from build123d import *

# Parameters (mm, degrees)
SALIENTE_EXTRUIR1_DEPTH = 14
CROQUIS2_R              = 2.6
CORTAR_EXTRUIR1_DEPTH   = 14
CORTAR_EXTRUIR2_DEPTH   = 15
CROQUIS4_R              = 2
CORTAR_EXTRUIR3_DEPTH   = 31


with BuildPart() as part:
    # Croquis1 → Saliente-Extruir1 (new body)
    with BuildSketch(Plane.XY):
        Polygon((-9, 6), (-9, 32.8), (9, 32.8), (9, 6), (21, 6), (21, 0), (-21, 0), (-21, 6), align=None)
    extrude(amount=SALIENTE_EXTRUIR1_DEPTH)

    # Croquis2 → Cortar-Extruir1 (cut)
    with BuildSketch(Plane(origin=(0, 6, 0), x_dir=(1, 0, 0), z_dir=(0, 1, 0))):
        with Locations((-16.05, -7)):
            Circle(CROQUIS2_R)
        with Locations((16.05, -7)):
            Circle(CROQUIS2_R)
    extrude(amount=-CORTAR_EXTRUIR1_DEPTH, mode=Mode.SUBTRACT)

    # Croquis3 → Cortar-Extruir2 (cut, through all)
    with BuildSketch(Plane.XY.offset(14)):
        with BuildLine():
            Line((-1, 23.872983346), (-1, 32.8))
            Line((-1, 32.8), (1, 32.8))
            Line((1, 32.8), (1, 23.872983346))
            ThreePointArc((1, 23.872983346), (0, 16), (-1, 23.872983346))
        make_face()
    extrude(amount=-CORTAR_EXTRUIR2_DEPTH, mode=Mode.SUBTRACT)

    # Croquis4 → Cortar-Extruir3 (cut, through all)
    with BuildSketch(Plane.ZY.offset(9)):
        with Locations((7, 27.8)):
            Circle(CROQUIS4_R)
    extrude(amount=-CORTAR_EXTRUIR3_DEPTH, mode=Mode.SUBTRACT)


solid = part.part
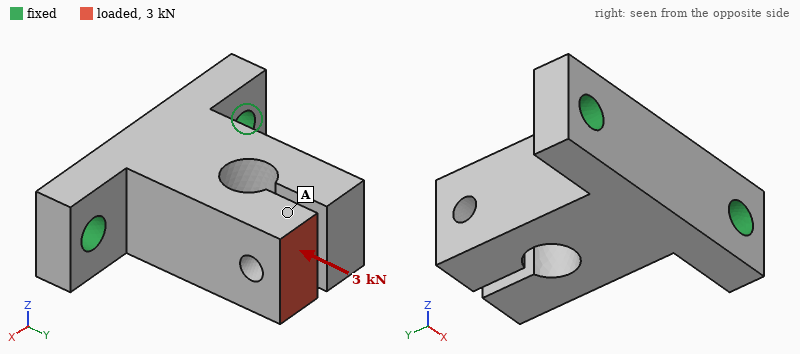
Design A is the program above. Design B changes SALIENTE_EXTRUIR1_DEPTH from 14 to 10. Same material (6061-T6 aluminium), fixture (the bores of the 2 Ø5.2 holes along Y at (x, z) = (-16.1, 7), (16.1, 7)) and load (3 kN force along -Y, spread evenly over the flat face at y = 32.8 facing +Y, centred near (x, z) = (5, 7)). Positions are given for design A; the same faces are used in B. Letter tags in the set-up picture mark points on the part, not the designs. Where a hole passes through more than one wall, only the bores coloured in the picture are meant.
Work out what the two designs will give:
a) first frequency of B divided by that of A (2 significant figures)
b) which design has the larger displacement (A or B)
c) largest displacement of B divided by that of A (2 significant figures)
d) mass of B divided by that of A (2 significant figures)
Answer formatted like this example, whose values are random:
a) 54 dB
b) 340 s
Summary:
a) 0.89
b) B
c) 1.5
d) 0.70
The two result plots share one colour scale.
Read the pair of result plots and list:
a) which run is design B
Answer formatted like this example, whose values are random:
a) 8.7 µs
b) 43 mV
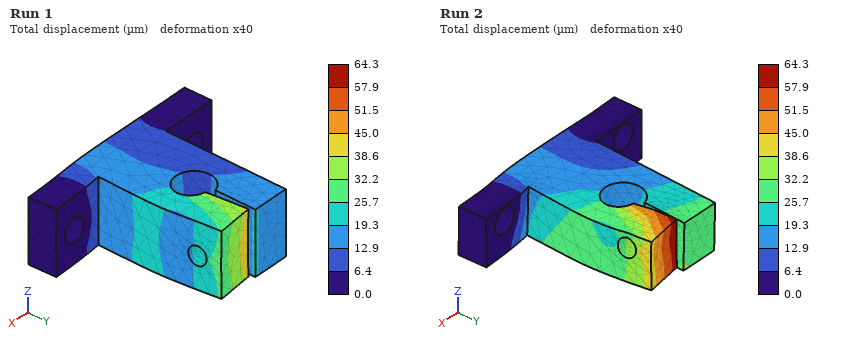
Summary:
a) Run 2
